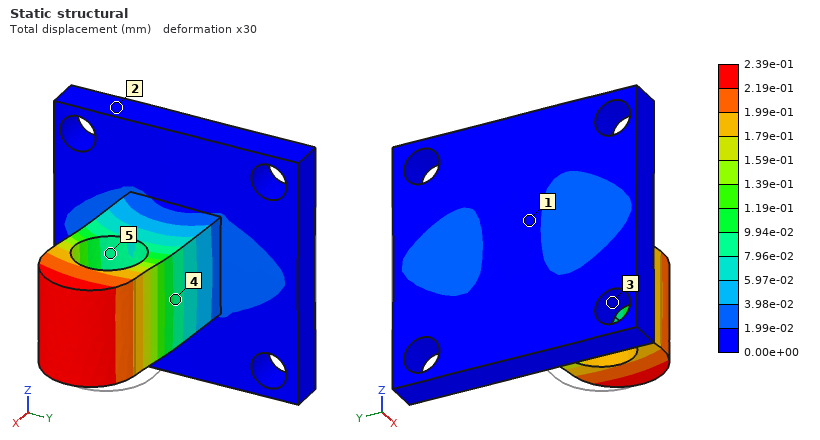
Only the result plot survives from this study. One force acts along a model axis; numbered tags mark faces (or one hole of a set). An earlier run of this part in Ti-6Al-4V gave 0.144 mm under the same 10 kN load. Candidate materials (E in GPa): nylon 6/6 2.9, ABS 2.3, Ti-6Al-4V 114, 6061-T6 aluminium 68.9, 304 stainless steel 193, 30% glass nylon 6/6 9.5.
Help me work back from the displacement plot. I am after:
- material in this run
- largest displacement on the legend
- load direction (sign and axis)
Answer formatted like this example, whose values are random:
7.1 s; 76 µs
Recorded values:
6061-T6 aluminium; 2.39e-01 mm; -Y
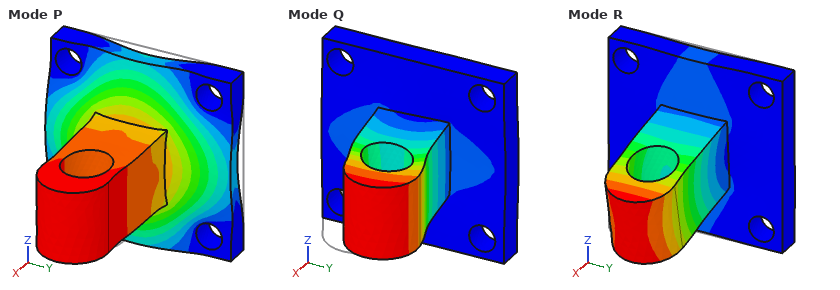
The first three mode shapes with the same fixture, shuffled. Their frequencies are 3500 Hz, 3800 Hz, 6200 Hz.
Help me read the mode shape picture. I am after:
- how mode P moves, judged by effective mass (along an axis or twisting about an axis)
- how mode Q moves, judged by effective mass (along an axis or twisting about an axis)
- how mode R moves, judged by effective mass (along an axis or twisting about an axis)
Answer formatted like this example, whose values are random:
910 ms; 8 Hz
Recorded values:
along X; along Y; along Z
